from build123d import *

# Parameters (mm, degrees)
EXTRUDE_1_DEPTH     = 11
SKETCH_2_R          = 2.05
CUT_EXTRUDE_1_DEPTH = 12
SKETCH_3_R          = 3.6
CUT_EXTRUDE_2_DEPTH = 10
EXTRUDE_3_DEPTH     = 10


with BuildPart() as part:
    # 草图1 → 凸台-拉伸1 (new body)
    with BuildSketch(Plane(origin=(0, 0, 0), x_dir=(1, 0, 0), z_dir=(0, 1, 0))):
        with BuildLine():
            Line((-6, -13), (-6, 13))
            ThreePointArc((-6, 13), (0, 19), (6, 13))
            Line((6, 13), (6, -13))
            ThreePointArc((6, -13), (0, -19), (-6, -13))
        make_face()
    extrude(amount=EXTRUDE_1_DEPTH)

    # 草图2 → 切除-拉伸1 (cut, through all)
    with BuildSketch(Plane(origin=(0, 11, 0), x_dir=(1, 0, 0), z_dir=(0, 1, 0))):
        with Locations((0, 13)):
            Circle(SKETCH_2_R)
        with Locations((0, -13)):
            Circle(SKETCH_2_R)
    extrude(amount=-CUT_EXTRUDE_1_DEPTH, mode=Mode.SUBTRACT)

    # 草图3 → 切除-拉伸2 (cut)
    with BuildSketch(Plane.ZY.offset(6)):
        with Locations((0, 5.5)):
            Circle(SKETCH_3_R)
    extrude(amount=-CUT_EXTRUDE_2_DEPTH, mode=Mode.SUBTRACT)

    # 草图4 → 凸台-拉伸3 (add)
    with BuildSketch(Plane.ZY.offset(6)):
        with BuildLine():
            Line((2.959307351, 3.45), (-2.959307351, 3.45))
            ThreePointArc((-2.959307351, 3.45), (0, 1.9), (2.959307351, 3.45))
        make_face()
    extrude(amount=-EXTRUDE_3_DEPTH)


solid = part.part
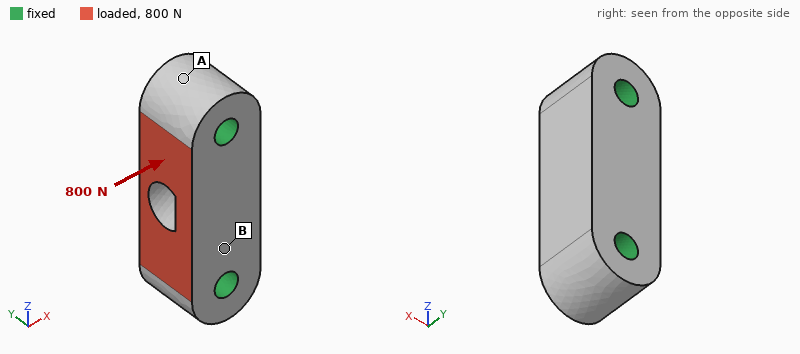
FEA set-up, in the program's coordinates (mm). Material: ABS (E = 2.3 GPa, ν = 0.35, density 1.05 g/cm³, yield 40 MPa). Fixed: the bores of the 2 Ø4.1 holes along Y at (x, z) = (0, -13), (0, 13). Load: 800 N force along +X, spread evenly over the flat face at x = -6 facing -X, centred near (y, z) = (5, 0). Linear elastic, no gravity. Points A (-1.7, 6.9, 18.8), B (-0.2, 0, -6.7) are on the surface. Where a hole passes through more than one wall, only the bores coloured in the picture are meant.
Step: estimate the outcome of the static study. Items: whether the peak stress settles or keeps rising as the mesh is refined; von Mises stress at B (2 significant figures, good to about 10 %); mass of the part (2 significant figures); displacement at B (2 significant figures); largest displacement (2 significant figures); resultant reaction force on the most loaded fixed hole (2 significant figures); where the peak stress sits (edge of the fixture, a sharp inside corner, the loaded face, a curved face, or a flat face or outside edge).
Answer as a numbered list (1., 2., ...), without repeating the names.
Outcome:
1. keeps rising
2. 4.5 MPa
3. 4.2 g
4. 27 µm
5. 50 µm
6. 400 N
7. edge of the fixture
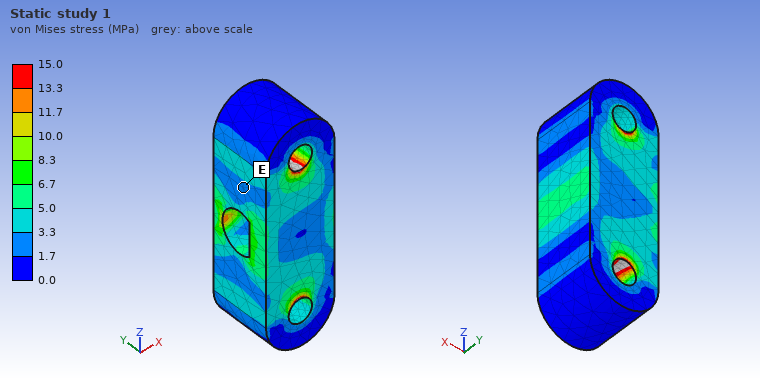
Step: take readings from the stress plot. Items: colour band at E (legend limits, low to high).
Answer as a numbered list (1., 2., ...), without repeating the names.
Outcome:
1. 1.7 to 3.3 MPa
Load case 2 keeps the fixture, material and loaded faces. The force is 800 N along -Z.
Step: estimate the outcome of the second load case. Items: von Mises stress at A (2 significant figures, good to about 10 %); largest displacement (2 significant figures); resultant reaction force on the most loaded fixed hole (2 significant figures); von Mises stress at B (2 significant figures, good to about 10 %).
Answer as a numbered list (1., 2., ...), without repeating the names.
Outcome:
1. 1.3 MPa
2. 31 µm
3. 420 N
4. 2.8 MPa
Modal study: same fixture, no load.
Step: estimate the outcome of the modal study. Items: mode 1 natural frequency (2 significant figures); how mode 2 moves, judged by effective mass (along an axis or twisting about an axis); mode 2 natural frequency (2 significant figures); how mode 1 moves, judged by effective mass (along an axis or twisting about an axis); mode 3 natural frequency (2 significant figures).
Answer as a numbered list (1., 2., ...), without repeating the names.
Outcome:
1. 14 kHz
2. along Y
3. 16 kHz
4. along X
5. 17 kHz
